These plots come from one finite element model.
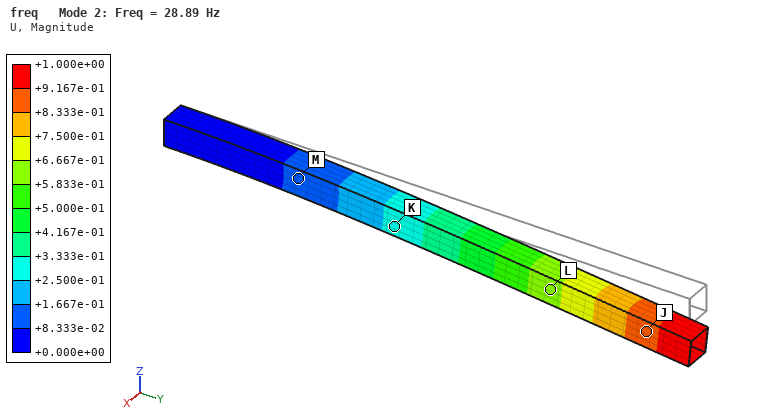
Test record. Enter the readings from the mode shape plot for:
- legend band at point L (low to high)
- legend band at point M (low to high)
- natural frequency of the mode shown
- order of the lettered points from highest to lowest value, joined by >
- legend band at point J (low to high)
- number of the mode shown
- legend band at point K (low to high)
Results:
+5.833e-01 to +6.667e-01
+8.333e-02 to +1.667e-01
28.89 Hz
J > L > K > M
+8.333e-01 to +9.167e-01
2
+2.500e-01 to +3.333e-01
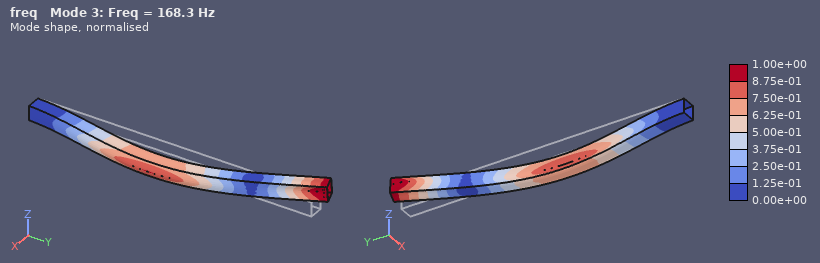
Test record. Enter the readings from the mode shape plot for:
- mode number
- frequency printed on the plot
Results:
3
168.3 Hz
